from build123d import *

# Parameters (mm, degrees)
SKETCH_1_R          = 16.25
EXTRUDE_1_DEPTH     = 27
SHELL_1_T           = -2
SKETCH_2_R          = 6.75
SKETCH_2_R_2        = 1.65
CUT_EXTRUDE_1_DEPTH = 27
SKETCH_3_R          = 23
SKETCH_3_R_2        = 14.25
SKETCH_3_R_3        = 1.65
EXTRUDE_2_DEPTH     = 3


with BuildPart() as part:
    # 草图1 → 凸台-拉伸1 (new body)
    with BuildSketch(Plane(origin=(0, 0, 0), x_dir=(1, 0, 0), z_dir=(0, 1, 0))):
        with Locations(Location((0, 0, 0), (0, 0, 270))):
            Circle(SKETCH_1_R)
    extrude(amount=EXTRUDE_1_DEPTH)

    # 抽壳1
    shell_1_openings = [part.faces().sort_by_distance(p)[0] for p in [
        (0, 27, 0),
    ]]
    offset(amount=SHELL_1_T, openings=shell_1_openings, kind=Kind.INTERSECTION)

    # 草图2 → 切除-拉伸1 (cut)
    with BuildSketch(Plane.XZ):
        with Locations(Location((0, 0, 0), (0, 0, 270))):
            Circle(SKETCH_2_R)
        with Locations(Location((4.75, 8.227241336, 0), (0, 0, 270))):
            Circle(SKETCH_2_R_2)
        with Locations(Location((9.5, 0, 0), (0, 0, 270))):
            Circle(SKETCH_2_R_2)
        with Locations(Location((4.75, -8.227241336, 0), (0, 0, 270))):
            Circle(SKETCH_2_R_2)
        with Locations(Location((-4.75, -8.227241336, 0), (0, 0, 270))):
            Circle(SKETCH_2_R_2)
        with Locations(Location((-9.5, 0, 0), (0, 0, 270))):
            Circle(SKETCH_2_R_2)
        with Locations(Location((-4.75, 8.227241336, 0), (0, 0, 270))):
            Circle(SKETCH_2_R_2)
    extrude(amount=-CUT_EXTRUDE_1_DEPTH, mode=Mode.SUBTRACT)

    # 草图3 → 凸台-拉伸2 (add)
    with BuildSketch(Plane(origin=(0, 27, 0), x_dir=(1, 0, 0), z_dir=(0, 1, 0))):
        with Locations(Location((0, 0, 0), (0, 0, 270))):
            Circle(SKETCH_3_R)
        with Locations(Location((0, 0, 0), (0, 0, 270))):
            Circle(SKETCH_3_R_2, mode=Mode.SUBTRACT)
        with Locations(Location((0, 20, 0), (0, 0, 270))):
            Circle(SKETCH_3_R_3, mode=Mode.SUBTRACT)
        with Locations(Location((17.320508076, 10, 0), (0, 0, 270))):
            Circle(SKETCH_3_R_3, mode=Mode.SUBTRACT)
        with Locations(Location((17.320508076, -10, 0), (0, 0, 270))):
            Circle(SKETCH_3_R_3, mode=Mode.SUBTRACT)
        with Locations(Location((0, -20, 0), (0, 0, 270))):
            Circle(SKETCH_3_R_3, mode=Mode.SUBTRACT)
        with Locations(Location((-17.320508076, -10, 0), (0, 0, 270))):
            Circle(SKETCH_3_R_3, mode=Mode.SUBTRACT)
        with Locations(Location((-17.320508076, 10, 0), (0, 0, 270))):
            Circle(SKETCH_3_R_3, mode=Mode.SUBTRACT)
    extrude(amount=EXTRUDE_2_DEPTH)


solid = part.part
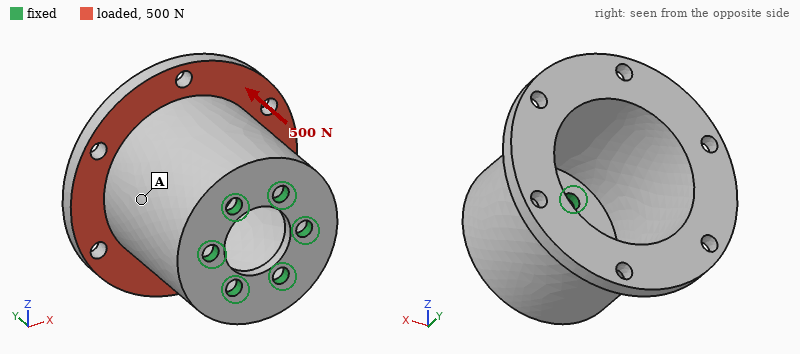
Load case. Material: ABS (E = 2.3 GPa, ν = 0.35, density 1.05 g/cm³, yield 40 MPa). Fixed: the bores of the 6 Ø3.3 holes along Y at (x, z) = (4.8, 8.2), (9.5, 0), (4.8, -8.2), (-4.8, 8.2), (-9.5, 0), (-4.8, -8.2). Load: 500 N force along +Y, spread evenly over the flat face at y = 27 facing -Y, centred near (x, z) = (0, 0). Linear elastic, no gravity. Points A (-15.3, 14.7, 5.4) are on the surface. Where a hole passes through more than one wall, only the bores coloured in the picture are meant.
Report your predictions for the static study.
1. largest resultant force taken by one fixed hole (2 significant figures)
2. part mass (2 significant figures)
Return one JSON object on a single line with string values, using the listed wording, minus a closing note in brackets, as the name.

{"largest resultant force taken by one fixed hole": "87 N", "part mass": "9.4 g"}
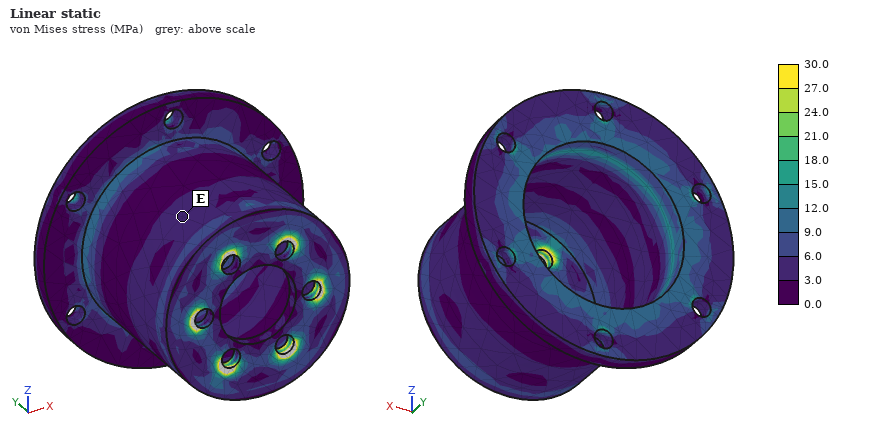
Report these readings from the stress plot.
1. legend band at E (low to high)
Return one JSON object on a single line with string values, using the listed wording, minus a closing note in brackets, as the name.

{"legend band at E": "3.0 to 6.0 MPa"}
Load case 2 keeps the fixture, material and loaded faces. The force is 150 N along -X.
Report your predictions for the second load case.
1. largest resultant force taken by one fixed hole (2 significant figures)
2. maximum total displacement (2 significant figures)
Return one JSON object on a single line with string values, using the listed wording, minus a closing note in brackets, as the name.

{"largest resultant force taken by one fixed hole": "95 N", "maximum total displacement": "0.39 mm"}
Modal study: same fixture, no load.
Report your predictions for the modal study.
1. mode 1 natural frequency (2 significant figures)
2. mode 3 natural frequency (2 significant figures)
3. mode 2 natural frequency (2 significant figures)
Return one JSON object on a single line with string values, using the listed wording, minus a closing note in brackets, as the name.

{"mode 1 natural frequency": "1400 Hz", "mode 3 natural frequency": "3500 Hz", "mode 2 natural frequency": "1400 Hz"}
